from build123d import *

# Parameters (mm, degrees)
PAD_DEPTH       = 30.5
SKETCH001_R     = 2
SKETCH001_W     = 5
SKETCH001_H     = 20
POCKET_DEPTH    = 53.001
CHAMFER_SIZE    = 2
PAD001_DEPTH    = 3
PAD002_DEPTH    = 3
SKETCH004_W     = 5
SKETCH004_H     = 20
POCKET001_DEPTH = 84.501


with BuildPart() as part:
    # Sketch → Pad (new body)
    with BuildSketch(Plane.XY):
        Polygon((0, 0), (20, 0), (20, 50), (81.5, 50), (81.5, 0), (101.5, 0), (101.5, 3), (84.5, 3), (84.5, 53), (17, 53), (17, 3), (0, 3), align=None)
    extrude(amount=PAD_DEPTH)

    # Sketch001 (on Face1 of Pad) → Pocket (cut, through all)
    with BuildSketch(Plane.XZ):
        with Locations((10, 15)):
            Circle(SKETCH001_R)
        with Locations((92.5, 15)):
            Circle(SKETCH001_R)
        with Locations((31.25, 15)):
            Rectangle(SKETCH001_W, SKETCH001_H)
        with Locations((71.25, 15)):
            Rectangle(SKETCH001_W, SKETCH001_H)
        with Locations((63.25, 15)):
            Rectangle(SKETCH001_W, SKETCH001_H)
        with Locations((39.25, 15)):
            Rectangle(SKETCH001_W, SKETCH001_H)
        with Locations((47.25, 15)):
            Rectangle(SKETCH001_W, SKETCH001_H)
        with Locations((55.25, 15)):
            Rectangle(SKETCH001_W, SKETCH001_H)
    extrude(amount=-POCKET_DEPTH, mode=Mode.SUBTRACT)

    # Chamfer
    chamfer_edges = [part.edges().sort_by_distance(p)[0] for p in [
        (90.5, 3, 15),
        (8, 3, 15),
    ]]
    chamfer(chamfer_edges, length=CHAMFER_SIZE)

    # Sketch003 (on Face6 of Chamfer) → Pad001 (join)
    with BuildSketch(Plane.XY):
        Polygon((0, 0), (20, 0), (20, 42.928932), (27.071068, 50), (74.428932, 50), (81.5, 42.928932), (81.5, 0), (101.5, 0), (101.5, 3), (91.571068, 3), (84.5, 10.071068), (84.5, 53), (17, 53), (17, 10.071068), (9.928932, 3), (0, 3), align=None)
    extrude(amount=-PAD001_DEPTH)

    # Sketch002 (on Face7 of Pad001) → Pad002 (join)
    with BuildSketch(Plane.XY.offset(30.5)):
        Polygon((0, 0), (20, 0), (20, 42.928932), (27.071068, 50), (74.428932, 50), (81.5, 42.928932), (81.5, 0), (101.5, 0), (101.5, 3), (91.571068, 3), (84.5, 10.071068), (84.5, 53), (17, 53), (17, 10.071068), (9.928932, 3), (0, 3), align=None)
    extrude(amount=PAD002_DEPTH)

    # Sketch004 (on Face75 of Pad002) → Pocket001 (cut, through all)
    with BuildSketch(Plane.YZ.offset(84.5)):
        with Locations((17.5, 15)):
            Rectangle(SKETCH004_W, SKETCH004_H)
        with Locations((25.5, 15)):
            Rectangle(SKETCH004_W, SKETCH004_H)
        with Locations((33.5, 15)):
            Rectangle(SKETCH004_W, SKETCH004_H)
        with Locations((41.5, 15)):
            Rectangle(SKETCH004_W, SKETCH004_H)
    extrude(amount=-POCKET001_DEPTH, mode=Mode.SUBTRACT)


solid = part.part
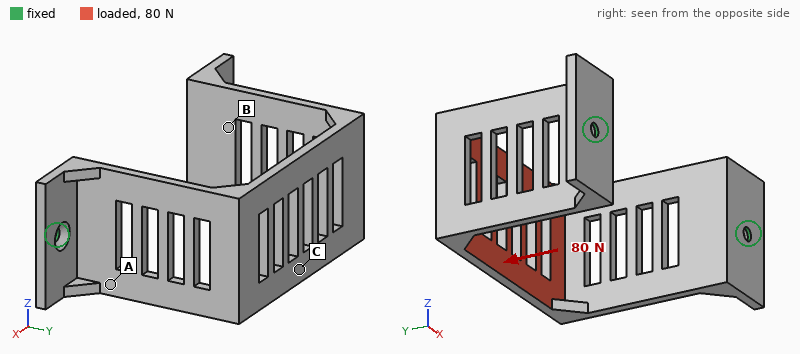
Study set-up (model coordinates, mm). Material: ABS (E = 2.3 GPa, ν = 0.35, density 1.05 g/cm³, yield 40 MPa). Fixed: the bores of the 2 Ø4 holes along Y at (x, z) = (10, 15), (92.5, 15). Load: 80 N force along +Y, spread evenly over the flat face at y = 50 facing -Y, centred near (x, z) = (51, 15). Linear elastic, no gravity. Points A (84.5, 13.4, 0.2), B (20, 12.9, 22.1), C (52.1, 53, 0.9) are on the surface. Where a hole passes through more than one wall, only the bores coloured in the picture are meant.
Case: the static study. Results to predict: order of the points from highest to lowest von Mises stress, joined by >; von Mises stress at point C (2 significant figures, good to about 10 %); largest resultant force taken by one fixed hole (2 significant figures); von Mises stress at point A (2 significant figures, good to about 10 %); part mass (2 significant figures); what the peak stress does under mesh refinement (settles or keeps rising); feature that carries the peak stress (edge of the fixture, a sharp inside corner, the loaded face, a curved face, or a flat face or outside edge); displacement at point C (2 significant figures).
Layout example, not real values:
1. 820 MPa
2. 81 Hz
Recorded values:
1. C > A > B
2. 9.9 MPa
3. 43 N
4. 4.6 MPa
5. 19 g
6. keeps rising
7. edge of the fixture
8. 0.95 mm
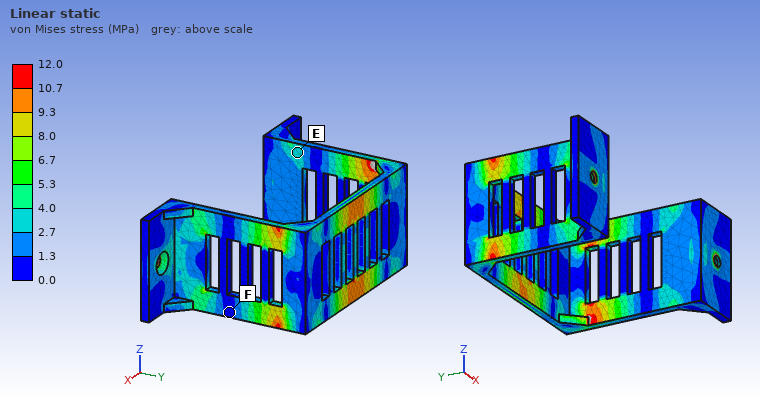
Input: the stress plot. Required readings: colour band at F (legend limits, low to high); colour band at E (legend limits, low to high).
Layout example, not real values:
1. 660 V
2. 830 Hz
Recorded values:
1. 0.0 to 1.3 MPa
2. 2.7 to 4.0 MPa
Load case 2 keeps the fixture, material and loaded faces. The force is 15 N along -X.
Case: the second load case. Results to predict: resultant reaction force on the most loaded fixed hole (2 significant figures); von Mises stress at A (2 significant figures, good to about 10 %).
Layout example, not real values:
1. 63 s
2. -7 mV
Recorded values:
1. 9.4 N
2. 3.3 MPa
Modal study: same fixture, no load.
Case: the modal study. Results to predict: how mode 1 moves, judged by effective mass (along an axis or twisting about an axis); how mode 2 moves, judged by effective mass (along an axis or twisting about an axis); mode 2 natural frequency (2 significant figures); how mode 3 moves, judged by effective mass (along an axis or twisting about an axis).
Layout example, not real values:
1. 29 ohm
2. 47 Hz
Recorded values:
1. along Z
2. along X
3. 190 Hz
4. twisting about Y
